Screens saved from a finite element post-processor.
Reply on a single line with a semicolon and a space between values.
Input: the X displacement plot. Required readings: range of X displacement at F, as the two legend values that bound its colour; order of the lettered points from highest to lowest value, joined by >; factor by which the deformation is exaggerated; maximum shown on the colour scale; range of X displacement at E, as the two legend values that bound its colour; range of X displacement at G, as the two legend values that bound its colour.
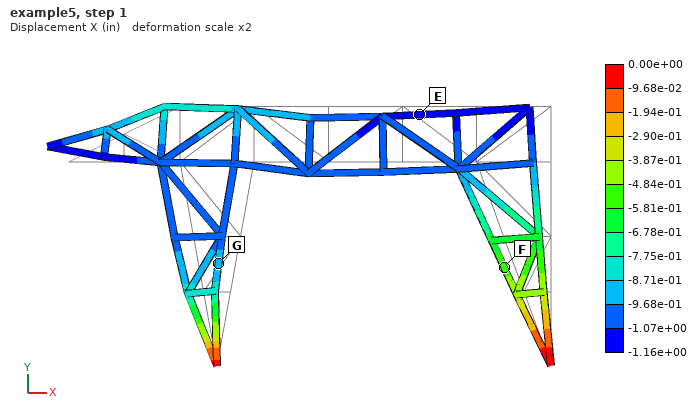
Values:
-5.81e-01 to -4.84e-01 in; F > G > E; 2; 0.00e+00 in; -1.16e+00 to -1.07e+00 in; -9.68e-01 to -8.71e-01 in
